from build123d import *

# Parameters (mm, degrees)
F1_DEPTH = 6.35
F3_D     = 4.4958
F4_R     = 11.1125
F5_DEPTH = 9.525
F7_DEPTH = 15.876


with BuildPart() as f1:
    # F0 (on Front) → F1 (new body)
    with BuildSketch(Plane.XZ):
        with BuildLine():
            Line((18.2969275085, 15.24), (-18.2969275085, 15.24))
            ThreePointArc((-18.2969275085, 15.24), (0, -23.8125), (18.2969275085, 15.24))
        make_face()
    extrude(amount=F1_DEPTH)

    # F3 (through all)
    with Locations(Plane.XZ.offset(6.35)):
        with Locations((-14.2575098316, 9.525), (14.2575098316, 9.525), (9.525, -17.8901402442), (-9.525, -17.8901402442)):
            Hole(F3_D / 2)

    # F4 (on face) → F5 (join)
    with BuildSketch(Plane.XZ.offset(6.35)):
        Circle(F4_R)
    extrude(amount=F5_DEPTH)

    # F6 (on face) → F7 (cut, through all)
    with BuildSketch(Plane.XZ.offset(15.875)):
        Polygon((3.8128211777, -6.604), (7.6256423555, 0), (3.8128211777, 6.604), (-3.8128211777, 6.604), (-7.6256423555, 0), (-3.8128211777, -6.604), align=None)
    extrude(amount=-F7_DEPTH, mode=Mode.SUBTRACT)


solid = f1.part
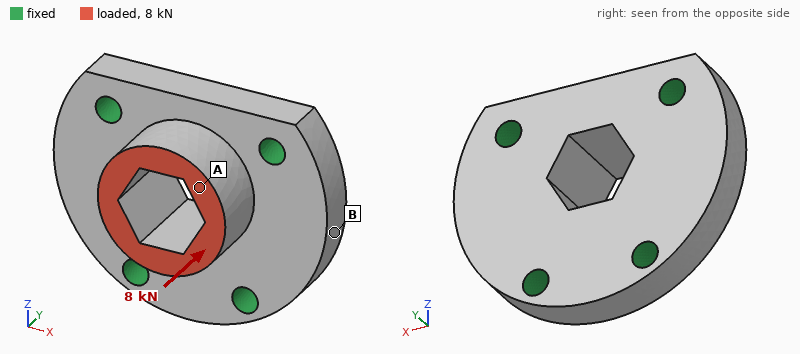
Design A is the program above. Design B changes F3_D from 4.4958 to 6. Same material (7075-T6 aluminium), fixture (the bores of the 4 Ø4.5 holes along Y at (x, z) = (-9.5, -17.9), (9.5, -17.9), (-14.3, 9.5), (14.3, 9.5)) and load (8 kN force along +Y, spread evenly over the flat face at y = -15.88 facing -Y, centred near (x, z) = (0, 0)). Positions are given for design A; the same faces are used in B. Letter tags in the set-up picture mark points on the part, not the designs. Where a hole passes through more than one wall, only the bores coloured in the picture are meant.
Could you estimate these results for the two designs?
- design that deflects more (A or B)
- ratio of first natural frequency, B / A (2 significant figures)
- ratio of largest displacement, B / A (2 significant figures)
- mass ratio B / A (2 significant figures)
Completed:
A
1.1
0.87
0.97
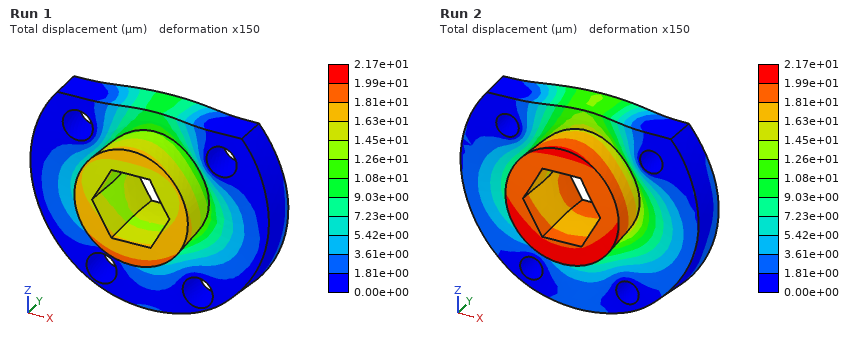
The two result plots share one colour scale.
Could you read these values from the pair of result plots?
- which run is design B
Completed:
Run 1
